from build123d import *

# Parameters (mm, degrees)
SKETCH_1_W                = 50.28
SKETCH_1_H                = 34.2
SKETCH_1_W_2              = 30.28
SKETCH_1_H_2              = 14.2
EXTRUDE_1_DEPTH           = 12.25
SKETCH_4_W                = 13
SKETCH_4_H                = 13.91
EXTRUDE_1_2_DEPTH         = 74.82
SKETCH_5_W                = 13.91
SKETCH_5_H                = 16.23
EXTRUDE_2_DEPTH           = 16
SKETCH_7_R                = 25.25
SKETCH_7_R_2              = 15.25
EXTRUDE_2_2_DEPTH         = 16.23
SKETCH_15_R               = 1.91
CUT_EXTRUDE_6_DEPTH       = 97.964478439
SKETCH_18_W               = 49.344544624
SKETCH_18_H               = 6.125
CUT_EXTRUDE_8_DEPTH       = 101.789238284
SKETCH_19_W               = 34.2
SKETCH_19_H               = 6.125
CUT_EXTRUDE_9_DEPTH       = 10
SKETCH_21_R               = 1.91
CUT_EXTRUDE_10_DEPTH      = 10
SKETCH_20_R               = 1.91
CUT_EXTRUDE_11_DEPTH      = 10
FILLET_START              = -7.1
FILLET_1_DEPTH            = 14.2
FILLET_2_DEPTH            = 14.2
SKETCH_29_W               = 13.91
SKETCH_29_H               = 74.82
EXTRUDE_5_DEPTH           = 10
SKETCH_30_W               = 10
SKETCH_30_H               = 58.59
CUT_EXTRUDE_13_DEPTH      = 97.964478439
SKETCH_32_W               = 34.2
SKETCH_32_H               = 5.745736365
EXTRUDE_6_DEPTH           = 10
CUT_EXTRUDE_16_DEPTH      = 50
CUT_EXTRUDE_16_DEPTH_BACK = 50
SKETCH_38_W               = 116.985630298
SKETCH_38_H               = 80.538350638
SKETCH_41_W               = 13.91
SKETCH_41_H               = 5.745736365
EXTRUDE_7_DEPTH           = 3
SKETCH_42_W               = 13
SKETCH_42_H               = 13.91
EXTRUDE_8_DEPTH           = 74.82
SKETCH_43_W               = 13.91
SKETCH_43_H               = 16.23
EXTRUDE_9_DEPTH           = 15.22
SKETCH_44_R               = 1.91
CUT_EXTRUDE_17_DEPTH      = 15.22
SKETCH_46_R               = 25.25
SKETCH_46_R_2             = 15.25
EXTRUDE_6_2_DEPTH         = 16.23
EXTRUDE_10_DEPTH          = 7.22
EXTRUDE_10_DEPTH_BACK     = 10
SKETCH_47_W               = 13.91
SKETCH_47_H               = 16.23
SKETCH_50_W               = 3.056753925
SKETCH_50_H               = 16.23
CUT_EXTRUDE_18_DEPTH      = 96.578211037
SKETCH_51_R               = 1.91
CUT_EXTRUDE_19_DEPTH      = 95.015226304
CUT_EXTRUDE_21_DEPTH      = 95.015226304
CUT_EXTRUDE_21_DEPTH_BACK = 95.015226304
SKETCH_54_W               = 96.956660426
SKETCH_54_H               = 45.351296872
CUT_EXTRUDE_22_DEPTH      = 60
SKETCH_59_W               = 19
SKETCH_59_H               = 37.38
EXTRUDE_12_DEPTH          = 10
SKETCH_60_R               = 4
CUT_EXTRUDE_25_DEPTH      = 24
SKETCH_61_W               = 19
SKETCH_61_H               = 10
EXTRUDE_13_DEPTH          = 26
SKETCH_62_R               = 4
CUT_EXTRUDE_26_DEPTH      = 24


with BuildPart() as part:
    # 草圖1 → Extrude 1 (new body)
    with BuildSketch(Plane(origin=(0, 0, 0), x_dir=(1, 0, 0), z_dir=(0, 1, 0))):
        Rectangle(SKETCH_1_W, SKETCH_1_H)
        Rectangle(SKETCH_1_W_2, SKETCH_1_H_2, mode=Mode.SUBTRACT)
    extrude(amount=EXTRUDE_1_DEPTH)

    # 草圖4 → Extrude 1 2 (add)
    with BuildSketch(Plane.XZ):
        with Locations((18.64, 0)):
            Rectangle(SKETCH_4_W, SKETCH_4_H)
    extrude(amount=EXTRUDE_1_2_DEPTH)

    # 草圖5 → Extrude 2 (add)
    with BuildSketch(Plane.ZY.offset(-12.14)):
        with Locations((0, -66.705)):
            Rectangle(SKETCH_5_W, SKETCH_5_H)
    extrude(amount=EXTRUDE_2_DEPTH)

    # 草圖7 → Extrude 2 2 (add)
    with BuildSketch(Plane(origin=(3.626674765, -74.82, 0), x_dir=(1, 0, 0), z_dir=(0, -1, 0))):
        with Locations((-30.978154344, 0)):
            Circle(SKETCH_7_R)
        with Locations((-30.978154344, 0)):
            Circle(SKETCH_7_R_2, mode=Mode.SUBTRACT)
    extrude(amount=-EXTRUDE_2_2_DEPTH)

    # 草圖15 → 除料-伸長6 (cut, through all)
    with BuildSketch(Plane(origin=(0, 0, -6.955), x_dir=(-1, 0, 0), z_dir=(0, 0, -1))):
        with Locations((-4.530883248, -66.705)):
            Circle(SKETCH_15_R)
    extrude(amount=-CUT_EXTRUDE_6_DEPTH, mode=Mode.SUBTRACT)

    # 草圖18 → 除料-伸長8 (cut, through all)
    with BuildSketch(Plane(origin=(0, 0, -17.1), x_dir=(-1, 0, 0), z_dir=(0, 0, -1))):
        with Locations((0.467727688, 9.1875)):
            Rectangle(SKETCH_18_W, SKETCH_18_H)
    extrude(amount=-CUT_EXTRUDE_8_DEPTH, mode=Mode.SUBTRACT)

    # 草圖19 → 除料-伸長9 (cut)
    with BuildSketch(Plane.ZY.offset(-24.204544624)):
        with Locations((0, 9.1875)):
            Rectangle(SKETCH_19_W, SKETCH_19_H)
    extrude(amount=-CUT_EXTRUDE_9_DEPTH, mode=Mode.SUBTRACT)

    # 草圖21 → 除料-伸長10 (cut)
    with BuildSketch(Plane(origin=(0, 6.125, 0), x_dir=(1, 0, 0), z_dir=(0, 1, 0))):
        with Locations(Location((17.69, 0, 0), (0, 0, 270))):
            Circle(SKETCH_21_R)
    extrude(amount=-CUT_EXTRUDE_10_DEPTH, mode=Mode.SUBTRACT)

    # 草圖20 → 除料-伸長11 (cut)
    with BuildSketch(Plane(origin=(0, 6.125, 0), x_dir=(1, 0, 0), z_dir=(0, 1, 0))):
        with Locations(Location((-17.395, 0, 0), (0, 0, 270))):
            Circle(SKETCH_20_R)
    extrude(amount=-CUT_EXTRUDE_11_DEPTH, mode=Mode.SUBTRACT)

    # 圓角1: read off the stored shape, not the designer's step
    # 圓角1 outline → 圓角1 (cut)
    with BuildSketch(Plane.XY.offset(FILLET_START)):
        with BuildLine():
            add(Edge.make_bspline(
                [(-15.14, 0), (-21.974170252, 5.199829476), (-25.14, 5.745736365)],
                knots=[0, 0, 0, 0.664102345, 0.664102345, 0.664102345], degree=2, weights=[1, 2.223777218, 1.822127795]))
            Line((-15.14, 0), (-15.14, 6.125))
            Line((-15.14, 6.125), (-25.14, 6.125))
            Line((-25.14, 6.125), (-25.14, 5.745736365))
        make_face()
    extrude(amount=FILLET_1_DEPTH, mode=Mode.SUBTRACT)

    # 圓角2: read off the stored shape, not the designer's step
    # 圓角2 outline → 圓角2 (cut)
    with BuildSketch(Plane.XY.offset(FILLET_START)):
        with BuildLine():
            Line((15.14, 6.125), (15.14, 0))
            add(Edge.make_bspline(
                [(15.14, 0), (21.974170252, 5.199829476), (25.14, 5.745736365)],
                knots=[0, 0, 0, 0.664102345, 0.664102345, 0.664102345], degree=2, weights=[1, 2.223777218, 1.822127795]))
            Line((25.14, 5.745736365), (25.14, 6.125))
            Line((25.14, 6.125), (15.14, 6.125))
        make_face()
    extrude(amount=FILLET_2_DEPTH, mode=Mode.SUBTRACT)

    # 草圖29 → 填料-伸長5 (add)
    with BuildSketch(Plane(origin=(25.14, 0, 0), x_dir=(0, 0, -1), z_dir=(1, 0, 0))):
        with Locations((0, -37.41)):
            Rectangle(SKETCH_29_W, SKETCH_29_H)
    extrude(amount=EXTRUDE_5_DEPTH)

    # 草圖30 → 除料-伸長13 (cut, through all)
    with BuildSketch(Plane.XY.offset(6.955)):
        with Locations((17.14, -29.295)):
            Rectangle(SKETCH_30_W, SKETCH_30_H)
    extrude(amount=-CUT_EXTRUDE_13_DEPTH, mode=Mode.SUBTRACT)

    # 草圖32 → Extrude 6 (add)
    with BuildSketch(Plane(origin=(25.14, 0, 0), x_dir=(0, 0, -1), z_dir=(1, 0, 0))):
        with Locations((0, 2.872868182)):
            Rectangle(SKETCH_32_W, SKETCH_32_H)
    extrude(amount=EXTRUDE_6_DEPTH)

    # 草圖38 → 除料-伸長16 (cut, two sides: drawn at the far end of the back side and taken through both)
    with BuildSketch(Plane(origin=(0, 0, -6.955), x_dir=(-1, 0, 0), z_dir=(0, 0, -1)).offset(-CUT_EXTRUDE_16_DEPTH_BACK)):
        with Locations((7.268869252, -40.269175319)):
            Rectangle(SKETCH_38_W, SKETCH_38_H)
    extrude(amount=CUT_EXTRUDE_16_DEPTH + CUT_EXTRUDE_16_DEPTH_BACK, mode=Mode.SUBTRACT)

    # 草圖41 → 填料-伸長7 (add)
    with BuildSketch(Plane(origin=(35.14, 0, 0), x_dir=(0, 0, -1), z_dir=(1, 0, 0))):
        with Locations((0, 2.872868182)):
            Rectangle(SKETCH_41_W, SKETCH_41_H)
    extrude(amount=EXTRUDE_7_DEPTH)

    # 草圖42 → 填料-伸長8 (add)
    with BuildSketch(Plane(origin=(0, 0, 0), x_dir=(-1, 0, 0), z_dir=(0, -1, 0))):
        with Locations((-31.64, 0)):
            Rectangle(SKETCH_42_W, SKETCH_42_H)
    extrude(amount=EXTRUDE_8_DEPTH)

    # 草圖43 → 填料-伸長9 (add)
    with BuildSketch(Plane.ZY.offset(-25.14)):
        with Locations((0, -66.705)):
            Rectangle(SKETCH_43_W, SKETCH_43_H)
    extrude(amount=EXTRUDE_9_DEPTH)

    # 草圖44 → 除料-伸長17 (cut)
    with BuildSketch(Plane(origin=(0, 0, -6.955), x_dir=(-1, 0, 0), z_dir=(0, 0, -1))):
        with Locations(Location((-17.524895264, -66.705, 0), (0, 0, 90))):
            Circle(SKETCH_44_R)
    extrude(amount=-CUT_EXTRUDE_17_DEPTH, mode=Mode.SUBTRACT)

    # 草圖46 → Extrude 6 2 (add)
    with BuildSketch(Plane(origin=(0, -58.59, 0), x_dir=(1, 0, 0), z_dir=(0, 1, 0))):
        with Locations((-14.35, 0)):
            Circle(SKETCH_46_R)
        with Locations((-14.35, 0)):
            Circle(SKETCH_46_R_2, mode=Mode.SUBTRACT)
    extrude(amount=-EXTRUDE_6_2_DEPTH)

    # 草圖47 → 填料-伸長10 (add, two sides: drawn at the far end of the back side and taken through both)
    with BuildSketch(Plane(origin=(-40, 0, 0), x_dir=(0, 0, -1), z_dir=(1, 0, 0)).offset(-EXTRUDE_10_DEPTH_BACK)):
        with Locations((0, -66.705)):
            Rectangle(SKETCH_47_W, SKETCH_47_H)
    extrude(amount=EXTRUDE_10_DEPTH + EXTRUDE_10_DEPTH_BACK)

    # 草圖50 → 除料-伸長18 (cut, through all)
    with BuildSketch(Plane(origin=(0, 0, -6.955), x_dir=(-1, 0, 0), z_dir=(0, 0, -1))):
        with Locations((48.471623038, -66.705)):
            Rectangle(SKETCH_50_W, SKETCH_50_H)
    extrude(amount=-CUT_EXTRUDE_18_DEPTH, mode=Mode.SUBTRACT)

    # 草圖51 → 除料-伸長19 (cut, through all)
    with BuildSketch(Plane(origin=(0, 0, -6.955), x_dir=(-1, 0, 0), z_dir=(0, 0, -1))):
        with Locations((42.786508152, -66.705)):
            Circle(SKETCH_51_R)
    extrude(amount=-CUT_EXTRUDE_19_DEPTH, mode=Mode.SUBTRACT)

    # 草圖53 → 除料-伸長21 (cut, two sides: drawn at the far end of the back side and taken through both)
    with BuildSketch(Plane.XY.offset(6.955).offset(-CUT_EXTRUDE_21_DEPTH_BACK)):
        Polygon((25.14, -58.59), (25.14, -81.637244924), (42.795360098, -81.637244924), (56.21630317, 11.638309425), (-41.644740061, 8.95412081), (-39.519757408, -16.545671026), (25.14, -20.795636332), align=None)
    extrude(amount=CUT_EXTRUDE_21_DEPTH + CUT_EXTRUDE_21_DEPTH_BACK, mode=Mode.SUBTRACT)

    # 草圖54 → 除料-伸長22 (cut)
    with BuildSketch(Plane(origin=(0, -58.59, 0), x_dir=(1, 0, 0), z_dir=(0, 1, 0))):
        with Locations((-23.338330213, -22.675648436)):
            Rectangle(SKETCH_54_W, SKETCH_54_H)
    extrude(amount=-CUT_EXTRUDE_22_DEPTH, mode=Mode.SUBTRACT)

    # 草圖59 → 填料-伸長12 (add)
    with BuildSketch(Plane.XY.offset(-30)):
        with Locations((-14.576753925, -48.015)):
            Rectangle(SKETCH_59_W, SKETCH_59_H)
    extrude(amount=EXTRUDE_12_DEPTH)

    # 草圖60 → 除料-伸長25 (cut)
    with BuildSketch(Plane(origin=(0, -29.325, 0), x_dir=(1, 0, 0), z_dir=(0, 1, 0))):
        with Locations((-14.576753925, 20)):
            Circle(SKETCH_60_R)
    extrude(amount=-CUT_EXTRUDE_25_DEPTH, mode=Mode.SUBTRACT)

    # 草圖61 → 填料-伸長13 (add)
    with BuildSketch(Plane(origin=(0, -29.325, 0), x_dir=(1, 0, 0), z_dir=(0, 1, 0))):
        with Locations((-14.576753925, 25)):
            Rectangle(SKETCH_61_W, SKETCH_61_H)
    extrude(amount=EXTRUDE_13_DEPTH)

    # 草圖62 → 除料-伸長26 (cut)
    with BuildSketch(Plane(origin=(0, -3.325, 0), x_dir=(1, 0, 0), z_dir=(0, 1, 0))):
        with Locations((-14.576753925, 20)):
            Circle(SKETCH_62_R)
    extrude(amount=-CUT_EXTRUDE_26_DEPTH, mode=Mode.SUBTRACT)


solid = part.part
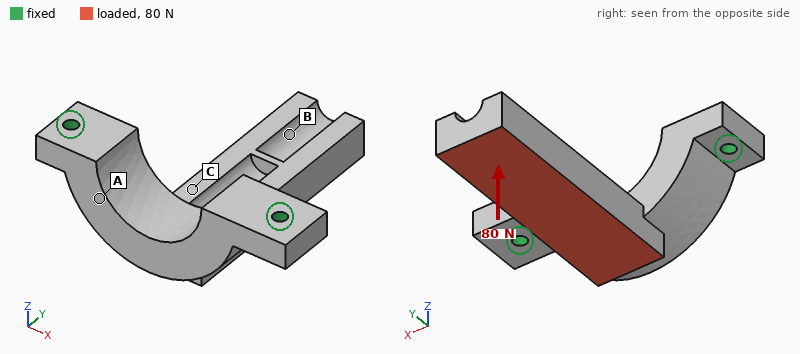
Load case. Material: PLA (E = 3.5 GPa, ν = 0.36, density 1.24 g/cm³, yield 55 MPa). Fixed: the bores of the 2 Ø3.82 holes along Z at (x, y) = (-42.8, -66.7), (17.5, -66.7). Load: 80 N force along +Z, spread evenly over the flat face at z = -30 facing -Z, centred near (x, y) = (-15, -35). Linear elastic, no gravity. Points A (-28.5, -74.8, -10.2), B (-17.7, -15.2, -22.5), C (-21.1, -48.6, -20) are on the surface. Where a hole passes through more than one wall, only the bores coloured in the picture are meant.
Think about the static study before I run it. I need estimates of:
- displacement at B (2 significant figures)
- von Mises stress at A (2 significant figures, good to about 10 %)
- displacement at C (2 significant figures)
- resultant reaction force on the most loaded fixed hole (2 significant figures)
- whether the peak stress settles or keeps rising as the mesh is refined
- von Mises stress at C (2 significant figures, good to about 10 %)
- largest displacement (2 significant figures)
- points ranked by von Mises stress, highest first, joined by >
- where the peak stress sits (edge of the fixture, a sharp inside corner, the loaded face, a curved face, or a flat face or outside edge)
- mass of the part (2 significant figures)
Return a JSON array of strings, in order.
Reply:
["0.84 mm", "3.1 MPa", "0.24 mm", "61 N", "keeps rising", "5.7 MPa", "1.1 mm", "C > A > B", "edge of the fixture", "28 g"]
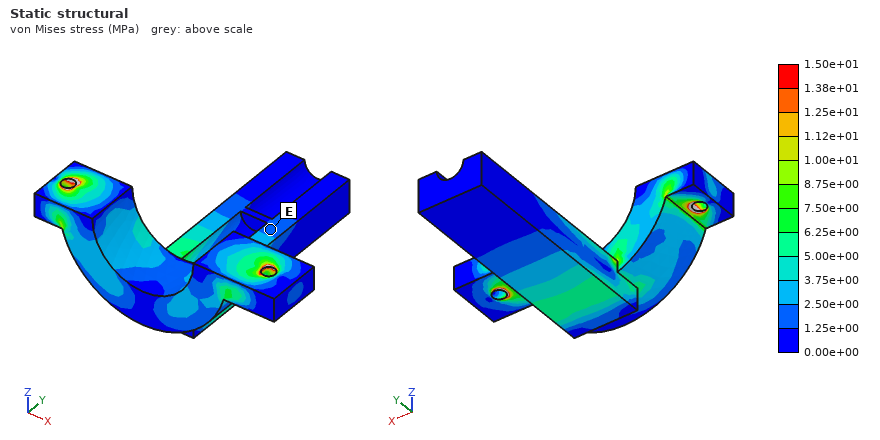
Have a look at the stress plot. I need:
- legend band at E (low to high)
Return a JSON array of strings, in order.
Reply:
["1.25e+00 to 2.50e+00 MPa"]
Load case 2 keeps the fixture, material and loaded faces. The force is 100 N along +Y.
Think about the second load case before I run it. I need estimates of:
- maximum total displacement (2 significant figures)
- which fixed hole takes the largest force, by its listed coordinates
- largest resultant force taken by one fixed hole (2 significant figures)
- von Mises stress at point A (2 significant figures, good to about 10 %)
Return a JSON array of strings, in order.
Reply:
["0.73 mm", "(-42.8, -66.7)", "56 N", "2.4 MPa"]
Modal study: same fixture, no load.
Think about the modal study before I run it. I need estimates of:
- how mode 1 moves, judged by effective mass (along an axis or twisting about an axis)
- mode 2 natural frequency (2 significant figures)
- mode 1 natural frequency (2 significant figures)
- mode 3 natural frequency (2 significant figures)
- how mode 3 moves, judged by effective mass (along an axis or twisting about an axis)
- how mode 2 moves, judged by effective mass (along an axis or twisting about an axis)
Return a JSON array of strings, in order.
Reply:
["along Z", "940 Hz", "440 Hz", "1300 Hz", "along Y", "along X"]
